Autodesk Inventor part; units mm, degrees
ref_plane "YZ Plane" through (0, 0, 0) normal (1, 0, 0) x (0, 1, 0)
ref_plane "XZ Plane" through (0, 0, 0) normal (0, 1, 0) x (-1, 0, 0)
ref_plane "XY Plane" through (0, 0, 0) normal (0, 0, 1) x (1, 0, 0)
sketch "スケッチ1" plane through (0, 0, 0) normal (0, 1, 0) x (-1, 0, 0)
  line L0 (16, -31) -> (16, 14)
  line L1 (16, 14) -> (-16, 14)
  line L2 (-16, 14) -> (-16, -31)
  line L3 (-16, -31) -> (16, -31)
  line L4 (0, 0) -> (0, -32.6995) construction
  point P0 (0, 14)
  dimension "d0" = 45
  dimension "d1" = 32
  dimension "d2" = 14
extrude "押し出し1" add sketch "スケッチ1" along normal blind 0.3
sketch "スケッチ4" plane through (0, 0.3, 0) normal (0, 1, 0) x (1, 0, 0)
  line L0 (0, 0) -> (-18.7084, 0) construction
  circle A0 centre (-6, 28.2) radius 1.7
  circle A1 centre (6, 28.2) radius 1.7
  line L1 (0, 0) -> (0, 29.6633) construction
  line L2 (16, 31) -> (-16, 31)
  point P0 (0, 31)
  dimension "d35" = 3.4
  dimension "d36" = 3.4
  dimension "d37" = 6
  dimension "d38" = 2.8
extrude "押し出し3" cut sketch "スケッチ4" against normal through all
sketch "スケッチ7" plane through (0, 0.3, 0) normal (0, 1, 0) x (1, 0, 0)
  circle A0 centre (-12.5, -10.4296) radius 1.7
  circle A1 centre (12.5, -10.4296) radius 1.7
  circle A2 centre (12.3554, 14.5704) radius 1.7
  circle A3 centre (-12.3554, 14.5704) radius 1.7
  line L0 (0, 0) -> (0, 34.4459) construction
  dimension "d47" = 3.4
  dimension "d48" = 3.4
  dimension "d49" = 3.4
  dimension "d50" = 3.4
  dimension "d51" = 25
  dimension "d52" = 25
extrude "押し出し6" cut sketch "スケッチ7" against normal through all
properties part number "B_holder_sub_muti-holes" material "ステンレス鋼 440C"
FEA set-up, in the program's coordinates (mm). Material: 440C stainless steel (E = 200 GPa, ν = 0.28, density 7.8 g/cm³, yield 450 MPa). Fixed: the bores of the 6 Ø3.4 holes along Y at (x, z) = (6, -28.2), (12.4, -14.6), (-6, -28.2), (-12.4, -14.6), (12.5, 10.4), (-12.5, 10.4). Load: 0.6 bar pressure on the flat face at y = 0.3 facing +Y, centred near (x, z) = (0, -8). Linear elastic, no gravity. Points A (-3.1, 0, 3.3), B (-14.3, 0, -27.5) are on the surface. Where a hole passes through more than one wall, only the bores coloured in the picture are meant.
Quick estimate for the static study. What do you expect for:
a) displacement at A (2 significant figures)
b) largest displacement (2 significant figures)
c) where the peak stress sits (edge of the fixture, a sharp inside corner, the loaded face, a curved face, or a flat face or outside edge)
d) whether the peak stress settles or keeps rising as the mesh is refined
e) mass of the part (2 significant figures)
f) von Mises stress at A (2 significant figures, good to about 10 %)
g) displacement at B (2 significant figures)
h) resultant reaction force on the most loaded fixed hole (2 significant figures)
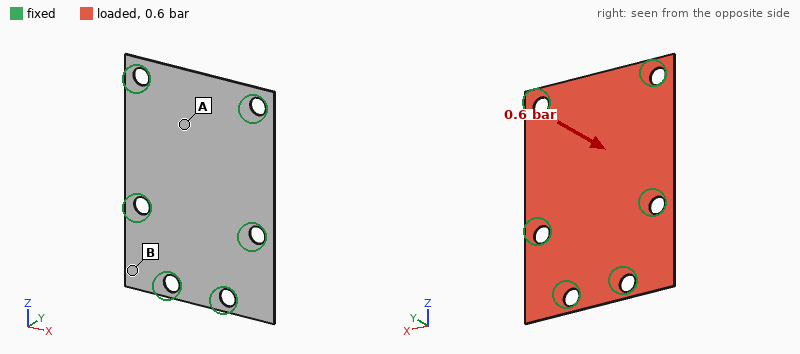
0.18 mm
0.23 mm
edge of the fixture
keeps rising
3.2 g
81 MPa
0.040 mm
18 N
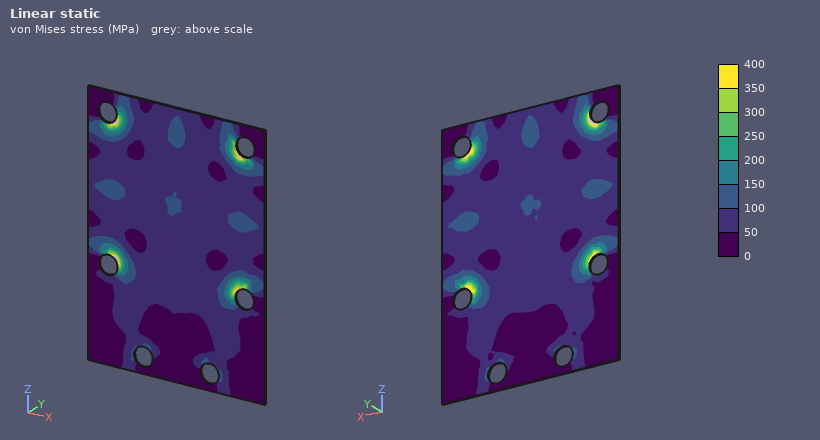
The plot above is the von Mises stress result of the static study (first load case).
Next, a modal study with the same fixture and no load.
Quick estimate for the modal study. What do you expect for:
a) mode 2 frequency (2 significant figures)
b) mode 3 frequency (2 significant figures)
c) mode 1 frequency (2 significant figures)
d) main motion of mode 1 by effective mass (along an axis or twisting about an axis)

3400 Hz
3500 Hz
2100 Hz
along Y
